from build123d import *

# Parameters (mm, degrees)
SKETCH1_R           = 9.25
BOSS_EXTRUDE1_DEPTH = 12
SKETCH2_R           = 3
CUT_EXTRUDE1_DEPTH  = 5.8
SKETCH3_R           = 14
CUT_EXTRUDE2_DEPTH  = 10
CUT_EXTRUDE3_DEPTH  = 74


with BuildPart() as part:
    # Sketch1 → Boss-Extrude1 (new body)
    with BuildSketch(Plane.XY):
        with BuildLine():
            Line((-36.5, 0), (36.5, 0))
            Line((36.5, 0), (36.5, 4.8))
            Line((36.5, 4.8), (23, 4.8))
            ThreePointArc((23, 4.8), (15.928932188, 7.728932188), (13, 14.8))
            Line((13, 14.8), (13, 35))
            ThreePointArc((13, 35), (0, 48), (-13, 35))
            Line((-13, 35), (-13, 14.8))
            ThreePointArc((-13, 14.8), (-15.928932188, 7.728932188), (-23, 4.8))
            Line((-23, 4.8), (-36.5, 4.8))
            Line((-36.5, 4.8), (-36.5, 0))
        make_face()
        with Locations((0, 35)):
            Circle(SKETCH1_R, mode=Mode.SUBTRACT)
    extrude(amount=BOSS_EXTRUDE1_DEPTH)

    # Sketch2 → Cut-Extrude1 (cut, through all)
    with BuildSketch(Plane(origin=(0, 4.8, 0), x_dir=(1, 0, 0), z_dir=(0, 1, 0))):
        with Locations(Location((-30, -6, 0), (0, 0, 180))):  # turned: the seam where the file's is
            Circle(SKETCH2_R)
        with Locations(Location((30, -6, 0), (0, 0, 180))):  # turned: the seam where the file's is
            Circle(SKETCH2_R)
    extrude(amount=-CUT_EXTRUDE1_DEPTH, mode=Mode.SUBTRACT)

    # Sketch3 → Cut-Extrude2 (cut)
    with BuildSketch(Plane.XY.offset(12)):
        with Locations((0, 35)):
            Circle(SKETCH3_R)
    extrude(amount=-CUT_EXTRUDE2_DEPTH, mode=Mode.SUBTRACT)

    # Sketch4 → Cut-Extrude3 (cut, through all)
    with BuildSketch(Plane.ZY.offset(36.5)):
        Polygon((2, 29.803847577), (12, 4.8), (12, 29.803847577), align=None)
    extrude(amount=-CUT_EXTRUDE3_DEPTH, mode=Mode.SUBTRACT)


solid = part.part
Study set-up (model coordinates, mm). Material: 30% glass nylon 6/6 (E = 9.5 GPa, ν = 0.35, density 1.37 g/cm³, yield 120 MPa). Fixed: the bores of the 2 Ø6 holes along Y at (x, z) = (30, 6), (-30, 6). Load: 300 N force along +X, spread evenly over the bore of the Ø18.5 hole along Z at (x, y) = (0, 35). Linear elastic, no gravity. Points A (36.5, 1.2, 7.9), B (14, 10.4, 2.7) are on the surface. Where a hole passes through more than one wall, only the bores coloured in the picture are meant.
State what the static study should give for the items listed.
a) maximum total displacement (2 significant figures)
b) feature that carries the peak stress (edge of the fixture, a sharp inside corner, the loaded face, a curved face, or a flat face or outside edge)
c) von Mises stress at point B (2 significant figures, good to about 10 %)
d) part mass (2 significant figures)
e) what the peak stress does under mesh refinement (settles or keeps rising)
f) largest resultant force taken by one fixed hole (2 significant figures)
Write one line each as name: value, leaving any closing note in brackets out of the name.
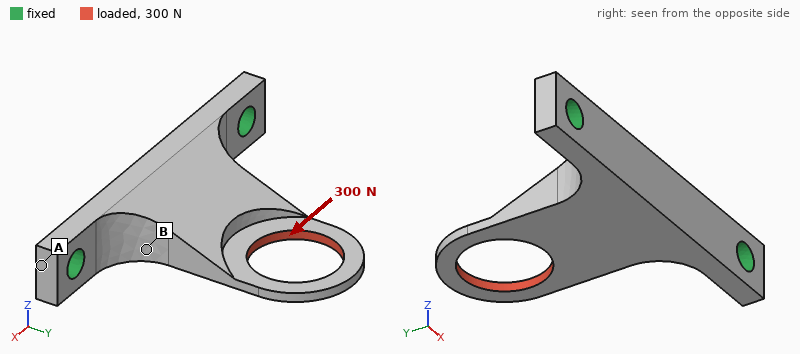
maximum total displacement: 0.48 mm
feature that carries the peak stress: a sharp inside corner
von Mises stress at point B: 15 MPa
part mass: 12 g
what the peak stress does under mesh refinement: keeps rising
largest resultant force taken by one fixed hole: 260 N
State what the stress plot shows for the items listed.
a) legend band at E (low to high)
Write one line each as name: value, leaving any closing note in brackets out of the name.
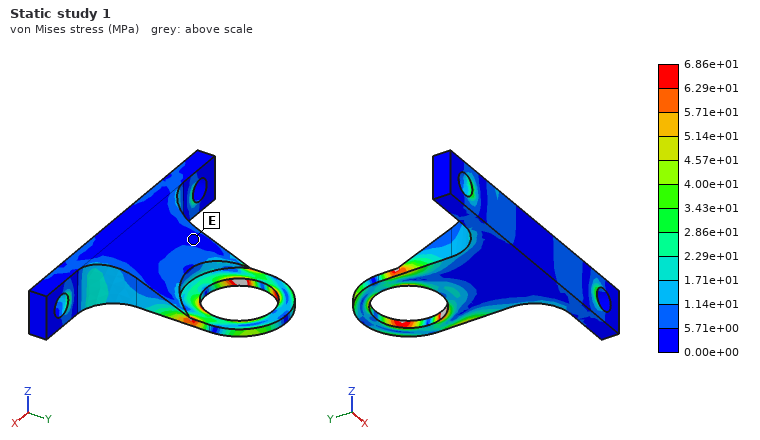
legend band at E: 0.00e+00 to 5.71e+00 MPa
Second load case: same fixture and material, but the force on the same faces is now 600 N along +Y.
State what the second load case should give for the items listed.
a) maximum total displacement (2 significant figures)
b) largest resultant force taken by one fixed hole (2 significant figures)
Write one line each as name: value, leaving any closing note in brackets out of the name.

maximum total displacement: 0.81 mm
largest resultant force taken by one fixed hole: 400 N
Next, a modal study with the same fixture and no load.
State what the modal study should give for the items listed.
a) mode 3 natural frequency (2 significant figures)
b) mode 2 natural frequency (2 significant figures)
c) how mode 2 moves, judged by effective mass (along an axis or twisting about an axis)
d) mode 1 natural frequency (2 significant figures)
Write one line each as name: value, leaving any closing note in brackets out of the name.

mode 3 natural frequency: 3800 Hz
mode 2 natural frequency: 2500 Hz
how mode 2 moves, judged by effective mass: along Z
mode 1 natural frequency: 1300 Hz
